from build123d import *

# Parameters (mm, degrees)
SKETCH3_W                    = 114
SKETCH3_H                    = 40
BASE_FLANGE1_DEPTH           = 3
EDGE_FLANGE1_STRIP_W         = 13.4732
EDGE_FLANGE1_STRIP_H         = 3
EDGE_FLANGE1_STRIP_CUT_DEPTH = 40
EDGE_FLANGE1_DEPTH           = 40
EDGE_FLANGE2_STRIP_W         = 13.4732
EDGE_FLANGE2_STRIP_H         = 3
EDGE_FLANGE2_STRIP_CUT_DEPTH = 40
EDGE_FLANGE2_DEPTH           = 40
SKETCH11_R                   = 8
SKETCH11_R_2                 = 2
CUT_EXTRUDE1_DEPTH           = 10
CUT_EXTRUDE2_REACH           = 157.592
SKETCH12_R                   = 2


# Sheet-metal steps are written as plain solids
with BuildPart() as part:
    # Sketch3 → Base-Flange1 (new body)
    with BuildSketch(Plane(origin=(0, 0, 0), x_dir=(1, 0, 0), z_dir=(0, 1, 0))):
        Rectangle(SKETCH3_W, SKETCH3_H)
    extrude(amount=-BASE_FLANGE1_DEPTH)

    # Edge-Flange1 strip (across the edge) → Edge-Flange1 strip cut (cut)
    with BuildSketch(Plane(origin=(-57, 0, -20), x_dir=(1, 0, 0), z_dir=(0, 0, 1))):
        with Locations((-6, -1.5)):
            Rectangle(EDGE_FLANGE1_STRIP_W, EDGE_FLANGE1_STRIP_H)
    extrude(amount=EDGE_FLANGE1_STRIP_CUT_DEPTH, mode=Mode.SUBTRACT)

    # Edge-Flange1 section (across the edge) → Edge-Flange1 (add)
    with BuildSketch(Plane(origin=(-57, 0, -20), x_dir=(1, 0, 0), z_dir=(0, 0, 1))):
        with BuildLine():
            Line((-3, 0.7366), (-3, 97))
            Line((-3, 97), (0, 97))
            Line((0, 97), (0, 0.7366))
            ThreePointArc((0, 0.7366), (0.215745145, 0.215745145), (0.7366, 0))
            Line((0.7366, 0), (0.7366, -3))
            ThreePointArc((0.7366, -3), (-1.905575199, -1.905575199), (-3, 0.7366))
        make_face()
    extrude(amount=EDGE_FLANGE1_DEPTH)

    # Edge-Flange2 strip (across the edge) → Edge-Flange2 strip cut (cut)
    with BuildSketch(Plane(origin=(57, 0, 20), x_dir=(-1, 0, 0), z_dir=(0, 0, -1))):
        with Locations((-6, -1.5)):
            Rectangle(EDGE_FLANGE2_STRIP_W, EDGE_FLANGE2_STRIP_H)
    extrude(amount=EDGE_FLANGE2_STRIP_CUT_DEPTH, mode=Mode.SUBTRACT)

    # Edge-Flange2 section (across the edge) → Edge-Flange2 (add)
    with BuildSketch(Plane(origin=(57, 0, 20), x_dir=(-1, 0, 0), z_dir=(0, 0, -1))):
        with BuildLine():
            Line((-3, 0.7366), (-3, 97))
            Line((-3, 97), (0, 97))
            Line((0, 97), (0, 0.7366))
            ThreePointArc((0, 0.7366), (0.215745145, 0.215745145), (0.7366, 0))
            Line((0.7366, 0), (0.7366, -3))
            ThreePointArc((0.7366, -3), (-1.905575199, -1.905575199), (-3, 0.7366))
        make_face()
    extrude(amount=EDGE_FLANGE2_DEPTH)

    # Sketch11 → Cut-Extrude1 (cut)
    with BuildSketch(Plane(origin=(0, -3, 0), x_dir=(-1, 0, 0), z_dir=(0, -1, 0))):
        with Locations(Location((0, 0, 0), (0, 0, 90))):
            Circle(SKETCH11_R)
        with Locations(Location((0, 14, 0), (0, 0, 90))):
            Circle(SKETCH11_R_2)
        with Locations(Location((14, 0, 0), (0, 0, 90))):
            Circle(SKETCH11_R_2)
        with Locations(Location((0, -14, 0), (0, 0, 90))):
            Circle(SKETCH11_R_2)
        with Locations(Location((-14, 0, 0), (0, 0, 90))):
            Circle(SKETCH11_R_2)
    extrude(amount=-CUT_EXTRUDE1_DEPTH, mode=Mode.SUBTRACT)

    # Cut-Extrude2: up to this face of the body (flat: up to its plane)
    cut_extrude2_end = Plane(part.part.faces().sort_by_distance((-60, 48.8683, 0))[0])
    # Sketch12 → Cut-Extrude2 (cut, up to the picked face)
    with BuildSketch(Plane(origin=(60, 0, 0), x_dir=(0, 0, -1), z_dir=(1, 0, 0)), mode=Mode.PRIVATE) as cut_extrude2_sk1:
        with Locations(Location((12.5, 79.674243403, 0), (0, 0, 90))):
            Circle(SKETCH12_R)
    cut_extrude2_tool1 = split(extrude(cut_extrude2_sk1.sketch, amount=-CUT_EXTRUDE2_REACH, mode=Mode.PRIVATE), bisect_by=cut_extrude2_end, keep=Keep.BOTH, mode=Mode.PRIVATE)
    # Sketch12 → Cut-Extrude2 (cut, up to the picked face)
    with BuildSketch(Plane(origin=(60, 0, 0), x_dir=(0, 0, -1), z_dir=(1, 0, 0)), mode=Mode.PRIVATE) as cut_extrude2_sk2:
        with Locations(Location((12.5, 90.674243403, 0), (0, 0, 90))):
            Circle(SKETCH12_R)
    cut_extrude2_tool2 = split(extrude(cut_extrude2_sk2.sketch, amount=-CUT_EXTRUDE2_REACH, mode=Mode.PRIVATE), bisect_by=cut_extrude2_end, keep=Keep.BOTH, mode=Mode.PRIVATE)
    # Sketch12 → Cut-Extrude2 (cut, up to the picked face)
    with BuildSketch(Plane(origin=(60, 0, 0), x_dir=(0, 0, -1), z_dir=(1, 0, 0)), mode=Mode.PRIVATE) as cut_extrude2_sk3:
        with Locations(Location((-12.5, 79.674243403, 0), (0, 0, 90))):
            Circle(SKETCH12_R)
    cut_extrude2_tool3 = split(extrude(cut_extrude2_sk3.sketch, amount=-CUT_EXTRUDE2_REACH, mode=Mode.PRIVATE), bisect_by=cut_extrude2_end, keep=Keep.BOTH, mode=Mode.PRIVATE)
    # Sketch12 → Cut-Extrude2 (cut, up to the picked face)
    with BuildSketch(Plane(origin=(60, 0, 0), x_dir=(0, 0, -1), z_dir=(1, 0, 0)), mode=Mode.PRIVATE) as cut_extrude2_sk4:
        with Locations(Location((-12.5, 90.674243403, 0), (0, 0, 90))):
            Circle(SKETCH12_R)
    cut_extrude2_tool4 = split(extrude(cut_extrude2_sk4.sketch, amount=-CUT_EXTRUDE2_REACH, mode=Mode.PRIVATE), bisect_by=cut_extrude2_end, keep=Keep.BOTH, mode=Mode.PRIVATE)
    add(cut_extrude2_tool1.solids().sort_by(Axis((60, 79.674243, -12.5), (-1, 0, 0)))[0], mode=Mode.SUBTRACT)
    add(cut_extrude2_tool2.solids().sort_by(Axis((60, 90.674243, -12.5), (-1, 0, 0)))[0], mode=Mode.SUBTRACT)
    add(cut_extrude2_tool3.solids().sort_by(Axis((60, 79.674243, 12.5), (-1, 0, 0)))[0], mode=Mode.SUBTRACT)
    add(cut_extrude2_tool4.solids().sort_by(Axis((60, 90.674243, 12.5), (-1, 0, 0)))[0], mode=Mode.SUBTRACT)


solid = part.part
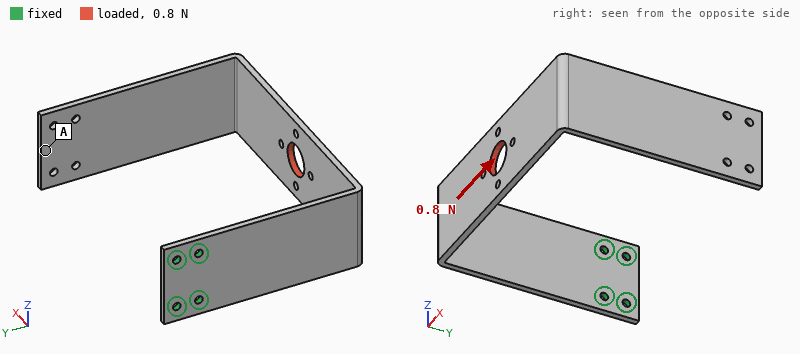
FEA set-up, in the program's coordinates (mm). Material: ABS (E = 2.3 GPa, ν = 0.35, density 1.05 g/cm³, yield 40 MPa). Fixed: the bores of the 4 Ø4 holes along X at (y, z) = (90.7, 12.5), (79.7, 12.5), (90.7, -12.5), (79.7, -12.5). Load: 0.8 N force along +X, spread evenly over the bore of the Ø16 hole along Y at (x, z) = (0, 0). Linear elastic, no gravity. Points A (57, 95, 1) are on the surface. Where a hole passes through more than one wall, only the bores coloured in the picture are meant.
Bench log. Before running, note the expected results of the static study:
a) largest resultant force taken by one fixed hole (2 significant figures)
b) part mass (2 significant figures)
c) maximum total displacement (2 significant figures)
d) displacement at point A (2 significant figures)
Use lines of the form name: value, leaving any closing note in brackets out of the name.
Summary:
largest resultant force taken by one fixed hole: 1.2 N
part mass: 38 g
maximum total displacement: 1.6 mm
displacement at point A: 1.5 mm
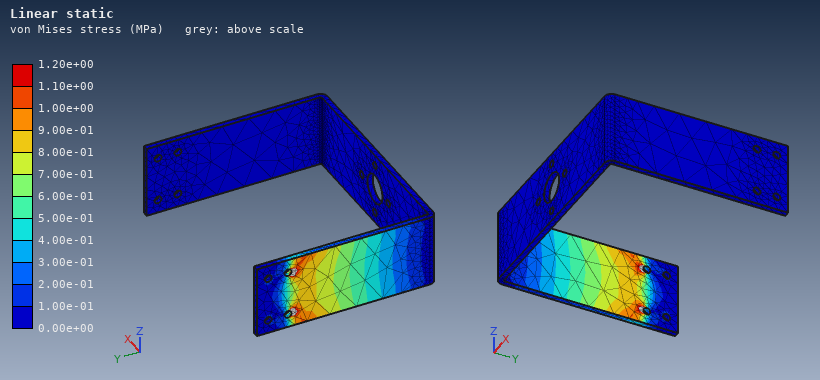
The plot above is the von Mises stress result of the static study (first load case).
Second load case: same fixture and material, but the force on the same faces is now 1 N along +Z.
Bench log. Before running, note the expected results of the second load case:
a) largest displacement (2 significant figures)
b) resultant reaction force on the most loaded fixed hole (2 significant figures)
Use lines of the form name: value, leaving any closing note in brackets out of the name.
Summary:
largest displacement: 1.7 mm
resultant reaction force on the most loaded fixed hole: 3.5 N
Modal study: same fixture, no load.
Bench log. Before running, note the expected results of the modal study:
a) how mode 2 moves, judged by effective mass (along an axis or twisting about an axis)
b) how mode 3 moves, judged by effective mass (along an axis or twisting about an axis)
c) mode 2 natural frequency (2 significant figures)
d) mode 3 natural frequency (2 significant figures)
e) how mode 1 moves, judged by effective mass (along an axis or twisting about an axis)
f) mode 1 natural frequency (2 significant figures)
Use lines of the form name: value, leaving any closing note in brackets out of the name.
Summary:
how mode 2 moves, judged by effective mass: along Z
how mode 3 moves, judged by effective mass: along X
mode 2 natural frequency: 20 Hz
mode 3 natural frequency: 33 Hz
how mode 1 moves, judged by effective mass: along Y
mode 1 natural frequency: 13 Hz
